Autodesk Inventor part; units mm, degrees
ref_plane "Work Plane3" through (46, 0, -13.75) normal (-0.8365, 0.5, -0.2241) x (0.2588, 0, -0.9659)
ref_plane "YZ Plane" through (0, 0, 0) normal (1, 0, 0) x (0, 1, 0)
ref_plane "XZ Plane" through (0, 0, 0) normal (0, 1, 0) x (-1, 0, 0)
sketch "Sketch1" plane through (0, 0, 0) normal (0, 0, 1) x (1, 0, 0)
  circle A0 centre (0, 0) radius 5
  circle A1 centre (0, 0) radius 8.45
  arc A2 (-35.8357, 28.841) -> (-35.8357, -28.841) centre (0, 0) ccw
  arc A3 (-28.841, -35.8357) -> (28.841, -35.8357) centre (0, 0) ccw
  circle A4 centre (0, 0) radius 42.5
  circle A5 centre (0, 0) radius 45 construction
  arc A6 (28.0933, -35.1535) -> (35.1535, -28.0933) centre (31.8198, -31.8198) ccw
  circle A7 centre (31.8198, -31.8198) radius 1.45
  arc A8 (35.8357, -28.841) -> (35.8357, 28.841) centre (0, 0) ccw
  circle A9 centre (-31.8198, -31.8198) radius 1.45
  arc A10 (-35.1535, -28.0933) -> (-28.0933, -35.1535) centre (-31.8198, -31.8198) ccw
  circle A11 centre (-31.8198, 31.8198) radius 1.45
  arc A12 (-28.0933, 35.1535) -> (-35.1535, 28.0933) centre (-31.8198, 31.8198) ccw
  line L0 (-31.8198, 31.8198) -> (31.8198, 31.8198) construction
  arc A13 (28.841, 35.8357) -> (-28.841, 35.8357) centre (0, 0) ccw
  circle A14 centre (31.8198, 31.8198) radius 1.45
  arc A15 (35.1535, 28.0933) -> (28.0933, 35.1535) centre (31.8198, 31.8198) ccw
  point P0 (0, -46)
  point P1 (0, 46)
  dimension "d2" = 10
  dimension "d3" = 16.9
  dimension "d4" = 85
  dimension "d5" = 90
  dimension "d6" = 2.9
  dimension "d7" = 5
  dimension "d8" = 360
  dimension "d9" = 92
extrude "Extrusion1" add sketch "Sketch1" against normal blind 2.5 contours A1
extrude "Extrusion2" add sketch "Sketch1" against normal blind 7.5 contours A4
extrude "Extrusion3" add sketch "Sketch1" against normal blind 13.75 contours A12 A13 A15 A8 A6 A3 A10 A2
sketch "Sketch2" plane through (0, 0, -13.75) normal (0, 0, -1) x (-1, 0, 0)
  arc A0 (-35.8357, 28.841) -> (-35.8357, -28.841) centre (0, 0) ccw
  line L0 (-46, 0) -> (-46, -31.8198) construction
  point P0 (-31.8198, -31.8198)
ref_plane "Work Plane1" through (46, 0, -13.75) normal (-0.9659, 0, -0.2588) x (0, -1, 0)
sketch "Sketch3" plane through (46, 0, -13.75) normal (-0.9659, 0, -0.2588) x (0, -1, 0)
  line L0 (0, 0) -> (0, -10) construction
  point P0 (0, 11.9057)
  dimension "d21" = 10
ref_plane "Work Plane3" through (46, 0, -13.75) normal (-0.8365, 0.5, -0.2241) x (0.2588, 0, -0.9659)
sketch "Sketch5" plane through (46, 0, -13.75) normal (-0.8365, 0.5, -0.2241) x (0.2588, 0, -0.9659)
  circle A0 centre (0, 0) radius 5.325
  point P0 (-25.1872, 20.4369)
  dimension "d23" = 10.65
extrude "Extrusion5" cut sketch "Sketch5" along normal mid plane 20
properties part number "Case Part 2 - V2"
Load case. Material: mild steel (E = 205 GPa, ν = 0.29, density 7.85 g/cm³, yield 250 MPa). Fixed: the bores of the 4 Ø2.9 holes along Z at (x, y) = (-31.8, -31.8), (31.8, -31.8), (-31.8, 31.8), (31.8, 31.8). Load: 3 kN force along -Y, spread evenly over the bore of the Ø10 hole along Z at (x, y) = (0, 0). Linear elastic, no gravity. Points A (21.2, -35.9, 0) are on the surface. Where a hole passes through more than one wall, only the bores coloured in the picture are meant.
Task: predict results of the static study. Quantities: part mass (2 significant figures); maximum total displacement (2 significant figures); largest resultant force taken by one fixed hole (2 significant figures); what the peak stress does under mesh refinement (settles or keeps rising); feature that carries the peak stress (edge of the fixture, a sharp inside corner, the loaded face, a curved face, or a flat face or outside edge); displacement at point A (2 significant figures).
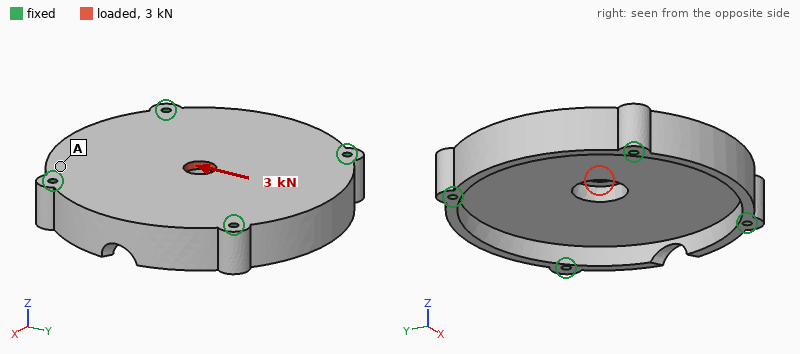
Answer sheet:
440 g
2.9 µm
790 N
keeps rising
a sharp inside corner
0.65 µm
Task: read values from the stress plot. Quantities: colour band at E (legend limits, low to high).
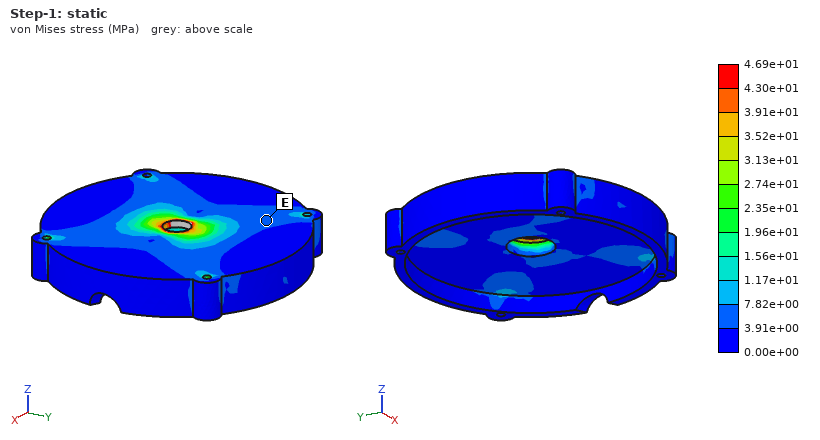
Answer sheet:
3.91e+00 to 7.82e+00 MPa
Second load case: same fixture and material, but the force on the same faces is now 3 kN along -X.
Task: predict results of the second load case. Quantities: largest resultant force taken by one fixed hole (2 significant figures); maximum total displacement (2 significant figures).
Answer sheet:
790 N
2.9 µm
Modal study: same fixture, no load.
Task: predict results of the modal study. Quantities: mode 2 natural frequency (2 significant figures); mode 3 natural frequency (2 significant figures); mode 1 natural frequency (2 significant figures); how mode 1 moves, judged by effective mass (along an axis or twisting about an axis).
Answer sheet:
9800 Hz
9900 Hz
6200 Hz
along Z
